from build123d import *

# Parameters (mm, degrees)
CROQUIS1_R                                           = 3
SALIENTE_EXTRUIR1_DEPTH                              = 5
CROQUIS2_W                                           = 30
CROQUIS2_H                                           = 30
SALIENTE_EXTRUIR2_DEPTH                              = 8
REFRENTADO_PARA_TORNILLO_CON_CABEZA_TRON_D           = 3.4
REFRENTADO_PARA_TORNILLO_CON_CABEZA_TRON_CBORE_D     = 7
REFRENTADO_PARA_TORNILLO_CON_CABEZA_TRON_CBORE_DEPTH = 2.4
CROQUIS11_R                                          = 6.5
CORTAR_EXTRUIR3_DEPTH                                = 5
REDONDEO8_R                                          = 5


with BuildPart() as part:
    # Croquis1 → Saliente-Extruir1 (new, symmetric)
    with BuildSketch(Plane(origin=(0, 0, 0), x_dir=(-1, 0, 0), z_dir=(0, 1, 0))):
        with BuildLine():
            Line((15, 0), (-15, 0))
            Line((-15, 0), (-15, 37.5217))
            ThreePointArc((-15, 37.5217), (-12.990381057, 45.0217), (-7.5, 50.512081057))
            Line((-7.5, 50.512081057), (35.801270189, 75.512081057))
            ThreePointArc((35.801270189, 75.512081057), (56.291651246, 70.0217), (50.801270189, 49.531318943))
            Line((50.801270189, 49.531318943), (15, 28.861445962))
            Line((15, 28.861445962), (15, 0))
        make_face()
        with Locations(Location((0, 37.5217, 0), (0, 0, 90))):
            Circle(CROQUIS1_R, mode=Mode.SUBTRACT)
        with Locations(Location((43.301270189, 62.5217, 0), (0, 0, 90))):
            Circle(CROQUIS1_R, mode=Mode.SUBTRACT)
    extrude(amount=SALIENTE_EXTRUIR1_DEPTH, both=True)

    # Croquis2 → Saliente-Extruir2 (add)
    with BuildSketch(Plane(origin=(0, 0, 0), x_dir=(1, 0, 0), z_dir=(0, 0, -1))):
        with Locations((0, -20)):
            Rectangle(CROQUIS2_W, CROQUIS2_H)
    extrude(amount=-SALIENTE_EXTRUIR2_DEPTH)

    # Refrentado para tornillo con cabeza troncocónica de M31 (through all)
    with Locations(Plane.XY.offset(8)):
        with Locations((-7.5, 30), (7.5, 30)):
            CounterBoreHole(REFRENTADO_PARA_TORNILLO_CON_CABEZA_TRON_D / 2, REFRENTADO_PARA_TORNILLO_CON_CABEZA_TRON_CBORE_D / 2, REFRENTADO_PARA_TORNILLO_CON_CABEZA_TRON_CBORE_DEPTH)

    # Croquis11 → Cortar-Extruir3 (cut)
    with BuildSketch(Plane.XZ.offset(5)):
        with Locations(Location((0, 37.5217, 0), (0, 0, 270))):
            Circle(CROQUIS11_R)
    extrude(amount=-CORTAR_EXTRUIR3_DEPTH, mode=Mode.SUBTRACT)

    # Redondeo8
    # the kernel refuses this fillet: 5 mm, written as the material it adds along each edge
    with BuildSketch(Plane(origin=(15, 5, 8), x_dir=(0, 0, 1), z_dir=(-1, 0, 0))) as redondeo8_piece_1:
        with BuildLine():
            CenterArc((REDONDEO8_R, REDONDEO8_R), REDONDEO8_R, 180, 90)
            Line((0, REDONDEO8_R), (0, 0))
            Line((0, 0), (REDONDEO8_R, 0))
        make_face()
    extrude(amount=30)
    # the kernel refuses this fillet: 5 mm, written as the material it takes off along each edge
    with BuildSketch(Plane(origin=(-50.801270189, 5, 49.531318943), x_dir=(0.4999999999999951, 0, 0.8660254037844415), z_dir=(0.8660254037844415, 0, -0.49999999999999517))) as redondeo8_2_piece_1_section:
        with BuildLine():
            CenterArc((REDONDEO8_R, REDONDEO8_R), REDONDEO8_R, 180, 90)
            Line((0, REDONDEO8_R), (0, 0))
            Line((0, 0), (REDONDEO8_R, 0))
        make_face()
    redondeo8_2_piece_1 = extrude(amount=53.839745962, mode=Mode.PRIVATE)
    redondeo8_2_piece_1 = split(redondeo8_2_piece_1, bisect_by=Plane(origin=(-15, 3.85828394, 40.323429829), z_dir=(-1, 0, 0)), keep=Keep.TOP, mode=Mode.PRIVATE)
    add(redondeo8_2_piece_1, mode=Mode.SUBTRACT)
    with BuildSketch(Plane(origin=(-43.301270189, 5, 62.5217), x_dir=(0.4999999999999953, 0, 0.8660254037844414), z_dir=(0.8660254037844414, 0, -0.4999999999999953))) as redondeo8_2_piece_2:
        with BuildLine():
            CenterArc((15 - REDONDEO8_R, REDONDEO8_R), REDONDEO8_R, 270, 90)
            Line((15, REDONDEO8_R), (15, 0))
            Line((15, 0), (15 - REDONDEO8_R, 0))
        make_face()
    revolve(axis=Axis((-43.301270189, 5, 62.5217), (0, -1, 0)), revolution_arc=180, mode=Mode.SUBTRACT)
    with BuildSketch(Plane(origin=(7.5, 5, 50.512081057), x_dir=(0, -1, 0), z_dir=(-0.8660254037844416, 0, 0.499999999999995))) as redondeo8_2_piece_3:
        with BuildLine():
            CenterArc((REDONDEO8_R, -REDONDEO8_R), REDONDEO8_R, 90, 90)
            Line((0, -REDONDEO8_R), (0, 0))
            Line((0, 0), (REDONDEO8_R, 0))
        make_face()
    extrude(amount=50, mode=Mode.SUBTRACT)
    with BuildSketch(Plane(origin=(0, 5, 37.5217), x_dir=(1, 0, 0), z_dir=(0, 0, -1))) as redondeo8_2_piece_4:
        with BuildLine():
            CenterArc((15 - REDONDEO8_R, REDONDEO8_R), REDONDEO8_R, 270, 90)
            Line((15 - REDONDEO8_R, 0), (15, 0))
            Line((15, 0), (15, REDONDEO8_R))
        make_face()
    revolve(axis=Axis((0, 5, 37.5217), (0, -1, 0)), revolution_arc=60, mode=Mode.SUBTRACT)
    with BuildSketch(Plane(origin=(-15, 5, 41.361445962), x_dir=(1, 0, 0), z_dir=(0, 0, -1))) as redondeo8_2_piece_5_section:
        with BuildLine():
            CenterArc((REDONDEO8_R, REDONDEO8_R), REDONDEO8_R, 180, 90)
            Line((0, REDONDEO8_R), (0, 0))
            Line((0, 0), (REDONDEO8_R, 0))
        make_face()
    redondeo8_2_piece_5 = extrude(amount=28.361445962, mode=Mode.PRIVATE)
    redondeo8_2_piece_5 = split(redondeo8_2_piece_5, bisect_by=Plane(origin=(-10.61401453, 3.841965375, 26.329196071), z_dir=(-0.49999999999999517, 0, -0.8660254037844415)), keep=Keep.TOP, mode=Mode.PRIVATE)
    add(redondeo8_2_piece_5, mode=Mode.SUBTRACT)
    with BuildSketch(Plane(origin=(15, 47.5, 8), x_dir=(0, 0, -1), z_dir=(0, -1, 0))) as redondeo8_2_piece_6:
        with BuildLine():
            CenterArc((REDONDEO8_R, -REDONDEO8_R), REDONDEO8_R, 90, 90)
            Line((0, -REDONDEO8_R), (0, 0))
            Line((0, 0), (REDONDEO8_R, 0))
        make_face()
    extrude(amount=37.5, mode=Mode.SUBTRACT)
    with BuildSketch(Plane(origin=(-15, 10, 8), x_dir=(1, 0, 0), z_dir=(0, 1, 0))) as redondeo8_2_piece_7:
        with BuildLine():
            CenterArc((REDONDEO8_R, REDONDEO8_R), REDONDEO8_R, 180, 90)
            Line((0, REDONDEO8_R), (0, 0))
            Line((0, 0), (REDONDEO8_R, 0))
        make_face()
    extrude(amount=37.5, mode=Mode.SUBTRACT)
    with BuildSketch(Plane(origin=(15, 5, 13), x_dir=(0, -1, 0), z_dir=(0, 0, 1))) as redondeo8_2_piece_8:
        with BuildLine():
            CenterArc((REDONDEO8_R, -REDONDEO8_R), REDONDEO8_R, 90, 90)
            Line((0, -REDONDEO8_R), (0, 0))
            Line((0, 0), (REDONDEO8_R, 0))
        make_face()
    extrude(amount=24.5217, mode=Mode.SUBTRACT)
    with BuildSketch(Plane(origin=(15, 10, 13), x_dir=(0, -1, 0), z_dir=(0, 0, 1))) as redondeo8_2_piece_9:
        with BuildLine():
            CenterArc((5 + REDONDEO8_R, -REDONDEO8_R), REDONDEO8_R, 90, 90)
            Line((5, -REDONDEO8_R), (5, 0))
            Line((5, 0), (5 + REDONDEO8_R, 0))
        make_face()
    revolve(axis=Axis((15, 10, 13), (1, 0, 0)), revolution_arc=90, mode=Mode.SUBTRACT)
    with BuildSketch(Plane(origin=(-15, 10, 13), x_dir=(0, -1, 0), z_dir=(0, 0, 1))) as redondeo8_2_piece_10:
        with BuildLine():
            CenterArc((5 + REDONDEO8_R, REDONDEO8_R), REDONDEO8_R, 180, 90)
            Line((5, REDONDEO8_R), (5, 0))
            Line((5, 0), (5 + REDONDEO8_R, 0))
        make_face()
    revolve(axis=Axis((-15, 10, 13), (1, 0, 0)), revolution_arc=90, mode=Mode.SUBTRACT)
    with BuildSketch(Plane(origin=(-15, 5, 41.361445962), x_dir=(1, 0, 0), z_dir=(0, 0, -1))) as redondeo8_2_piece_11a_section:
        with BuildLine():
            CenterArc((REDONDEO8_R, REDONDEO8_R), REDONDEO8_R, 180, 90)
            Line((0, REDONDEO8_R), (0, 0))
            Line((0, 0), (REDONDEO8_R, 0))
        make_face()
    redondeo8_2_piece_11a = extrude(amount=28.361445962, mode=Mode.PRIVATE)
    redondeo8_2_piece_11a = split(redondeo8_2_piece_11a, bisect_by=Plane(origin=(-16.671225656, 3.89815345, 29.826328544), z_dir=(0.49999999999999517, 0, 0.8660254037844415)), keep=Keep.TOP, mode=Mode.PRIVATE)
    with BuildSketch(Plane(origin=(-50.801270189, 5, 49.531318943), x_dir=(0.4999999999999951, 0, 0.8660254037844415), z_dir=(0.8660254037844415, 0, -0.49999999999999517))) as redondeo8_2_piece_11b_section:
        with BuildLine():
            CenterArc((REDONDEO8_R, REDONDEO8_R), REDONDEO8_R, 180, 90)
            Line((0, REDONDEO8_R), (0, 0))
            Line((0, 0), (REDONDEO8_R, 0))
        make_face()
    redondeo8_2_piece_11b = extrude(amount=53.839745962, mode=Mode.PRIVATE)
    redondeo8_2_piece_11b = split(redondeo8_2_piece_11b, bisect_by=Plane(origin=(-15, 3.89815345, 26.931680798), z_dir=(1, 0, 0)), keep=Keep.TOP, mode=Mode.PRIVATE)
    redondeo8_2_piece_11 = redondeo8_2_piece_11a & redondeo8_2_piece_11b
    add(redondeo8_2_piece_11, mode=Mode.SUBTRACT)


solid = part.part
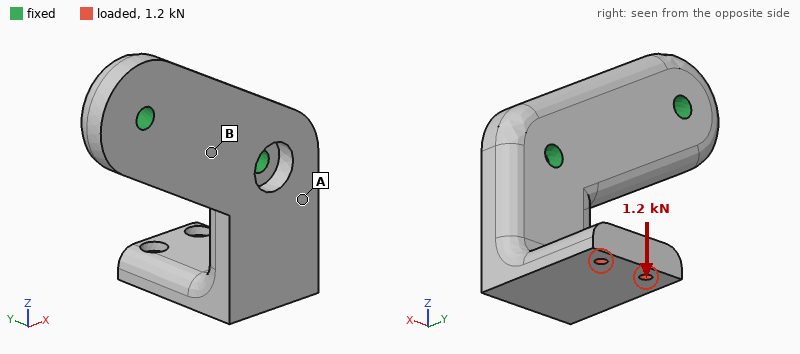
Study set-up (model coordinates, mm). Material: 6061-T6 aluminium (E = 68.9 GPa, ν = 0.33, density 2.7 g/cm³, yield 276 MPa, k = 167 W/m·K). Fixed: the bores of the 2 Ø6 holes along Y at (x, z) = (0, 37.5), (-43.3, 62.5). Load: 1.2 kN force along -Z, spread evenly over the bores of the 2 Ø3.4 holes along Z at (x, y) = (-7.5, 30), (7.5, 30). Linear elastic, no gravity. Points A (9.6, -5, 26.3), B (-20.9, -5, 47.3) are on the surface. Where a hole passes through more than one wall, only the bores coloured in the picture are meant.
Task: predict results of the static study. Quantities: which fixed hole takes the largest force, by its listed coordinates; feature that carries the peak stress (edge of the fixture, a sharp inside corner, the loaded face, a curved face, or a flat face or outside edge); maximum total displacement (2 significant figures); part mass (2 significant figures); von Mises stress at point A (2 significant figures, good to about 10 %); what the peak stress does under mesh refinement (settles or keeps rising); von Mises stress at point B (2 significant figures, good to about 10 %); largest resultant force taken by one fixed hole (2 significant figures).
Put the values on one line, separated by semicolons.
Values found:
(0, 37.5); edge of the fixture; 0.49 mm; 93 g; 74 MPa; keeps rising; 20 MPa; 1.5 kN
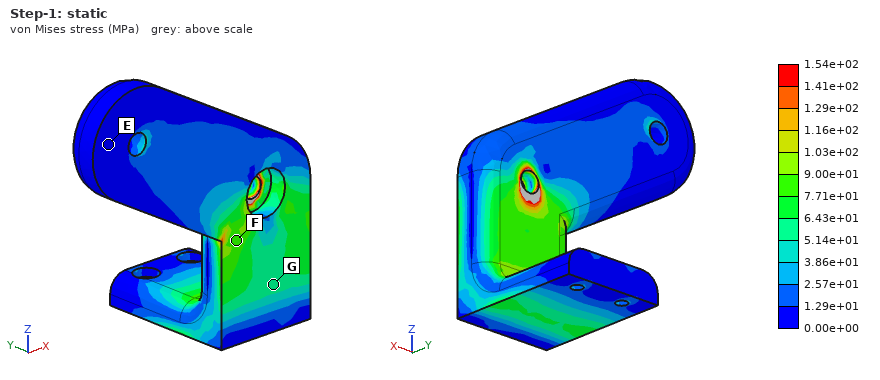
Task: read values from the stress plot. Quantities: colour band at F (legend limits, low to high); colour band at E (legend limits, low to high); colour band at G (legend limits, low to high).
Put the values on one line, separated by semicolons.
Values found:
7.71e+01 to 9.00e+01 MPa; 0.00e+00 to 1.29e+01 MPa; 5.14e+01 to 6.43e+01 MPa
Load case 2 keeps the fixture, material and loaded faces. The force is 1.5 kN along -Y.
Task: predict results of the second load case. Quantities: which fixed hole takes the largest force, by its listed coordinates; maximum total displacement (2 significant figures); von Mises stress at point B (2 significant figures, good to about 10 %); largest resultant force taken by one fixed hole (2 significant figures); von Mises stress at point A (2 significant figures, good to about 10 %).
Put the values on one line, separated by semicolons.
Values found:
(0, 37.5); 0.43 mm; 32 MPa; 2.0 kN; 76 MPa
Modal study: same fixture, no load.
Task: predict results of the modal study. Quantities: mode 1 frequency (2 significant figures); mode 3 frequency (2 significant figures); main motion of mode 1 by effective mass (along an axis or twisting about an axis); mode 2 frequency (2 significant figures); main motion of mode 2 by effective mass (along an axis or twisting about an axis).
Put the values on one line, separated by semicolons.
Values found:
2000 Hz; 5800 Hz; along Y; 3300 Hz; along X
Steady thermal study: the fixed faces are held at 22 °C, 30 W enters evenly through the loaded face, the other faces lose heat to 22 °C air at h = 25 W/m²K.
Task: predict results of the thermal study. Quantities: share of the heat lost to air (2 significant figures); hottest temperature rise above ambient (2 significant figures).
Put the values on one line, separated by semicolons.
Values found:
11 %; 44 K
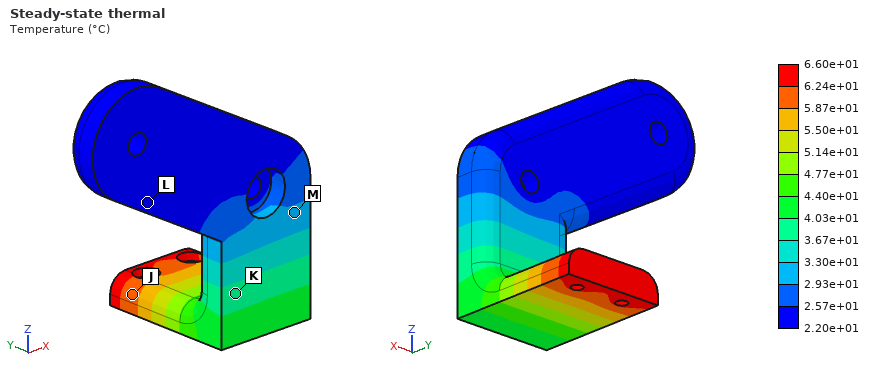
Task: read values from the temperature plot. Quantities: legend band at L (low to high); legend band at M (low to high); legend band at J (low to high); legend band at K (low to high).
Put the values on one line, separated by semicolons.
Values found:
2.20e+01 to 2.57e+01 °C; 2.93e+01 to 3.30e+01 °C; 5.87e+01 to 6.24e+01 °C; 3.67e+01 to 4.03e+01 °C
